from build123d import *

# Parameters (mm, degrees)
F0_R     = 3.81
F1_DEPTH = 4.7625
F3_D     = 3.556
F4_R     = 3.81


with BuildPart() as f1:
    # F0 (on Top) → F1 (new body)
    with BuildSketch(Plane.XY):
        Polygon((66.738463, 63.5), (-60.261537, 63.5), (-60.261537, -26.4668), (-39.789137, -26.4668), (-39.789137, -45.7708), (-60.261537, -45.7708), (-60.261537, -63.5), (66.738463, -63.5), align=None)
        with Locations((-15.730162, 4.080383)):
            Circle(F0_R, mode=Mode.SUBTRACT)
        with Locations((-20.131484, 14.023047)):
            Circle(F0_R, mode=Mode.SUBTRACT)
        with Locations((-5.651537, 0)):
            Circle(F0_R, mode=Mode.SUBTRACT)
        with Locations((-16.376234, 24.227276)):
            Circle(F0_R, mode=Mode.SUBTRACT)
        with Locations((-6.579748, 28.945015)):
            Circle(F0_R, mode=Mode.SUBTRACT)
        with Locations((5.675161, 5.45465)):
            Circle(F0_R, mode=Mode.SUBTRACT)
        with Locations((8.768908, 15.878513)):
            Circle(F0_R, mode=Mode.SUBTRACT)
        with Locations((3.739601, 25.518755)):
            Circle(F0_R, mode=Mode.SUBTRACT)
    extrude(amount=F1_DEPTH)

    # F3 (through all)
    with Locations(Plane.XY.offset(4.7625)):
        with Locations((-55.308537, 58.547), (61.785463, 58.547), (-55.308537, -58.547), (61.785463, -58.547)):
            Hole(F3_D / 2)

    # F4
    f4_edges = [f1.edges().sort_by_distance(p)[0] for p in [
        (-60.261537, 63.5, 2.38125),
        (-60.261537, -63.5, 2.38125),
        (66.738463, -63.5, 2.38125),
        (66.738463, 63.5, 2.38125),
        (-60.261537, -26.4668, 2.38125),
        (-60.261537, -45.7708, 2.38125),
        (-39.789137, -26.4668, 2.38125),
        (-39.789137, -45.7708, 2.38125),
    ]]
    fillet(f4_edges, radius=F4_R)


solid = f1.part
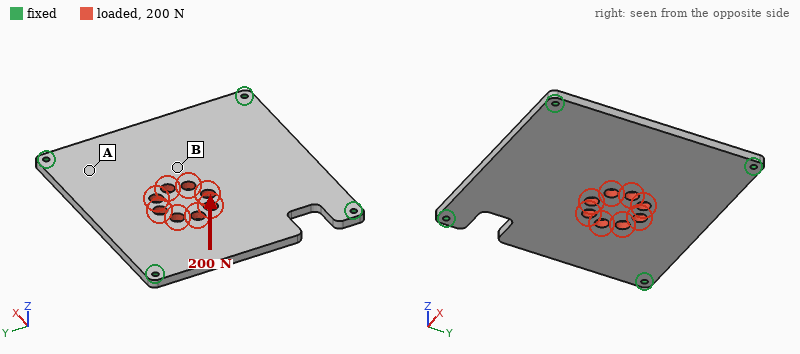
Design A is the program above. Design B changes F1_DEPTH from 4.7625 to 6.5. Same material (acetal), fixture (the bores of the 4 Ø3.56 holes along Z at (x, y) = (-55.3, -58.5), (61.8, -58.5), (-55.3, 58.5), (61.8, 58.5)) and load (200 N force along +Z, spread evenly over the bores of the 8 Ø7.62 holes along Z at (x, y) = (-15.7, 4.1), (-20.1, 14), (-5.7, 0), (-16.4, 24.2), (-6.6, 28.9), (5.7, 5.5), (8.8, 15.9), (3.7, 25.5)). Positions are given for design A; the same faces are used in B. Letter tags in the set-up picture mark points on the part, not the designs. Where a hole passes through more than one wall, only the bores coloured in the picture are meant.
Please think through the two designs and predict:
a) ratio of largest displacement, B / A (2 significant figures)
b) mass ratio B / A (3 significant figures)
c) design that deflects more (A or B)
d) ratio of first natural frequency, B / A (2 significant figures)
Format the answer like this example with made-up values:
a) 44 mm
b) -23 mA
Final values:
a) 0.41
b) 1.36
c) A
d) 1.3
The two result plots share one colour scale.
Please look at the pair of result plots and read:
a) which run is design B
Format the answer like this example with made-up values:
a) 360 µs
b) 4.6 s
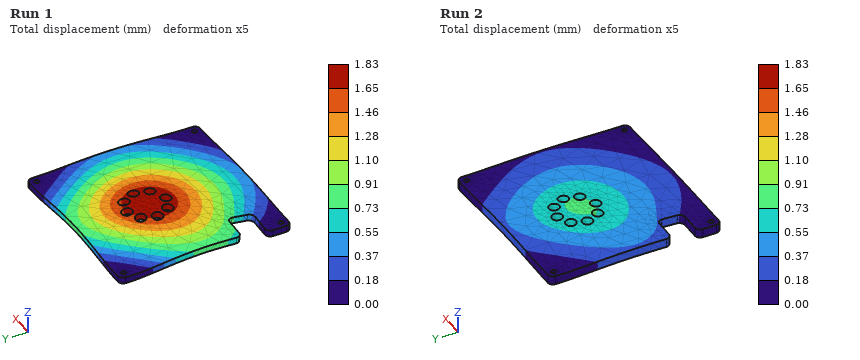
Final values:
a) Run 2
